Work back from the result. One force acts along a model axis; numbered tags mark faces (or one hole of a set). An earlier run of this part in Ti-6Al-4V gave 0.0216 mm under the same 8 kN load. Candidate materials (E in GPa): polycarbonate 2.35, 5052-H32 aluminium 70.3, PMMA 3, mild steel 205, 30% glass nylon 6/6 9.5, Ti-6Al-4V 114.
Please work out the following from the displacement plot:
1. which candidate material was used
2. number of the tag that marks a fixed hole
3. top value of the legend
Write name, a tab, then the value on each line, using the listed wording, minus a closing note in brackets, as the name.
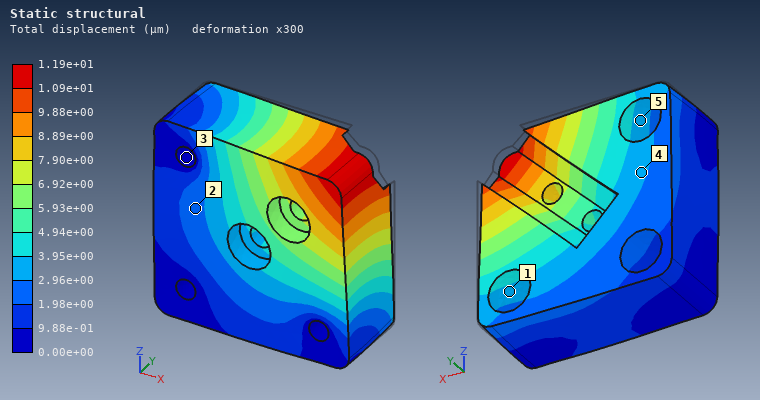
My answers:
which candidate material was used	mild steel
number of the tag that marks a fixed hole	3
top value of the legend	1.19e+01 µm
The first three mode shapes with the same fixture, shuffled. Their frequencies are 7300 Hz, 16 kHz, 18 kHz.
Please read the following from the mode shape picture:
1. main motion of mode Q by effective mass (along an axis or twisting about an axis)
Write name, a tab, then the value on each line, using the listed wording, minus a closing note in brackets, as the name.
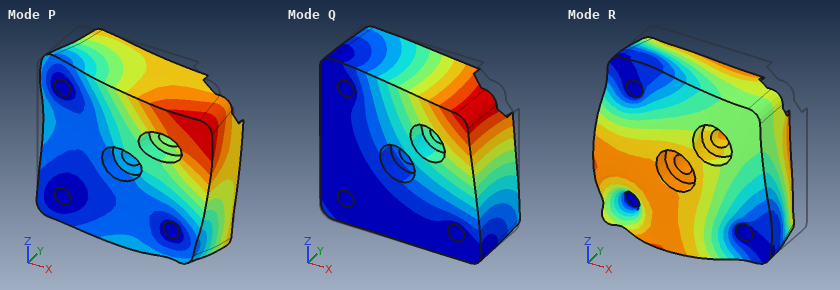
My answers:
main motion of mode Q by effective mass	along Y
